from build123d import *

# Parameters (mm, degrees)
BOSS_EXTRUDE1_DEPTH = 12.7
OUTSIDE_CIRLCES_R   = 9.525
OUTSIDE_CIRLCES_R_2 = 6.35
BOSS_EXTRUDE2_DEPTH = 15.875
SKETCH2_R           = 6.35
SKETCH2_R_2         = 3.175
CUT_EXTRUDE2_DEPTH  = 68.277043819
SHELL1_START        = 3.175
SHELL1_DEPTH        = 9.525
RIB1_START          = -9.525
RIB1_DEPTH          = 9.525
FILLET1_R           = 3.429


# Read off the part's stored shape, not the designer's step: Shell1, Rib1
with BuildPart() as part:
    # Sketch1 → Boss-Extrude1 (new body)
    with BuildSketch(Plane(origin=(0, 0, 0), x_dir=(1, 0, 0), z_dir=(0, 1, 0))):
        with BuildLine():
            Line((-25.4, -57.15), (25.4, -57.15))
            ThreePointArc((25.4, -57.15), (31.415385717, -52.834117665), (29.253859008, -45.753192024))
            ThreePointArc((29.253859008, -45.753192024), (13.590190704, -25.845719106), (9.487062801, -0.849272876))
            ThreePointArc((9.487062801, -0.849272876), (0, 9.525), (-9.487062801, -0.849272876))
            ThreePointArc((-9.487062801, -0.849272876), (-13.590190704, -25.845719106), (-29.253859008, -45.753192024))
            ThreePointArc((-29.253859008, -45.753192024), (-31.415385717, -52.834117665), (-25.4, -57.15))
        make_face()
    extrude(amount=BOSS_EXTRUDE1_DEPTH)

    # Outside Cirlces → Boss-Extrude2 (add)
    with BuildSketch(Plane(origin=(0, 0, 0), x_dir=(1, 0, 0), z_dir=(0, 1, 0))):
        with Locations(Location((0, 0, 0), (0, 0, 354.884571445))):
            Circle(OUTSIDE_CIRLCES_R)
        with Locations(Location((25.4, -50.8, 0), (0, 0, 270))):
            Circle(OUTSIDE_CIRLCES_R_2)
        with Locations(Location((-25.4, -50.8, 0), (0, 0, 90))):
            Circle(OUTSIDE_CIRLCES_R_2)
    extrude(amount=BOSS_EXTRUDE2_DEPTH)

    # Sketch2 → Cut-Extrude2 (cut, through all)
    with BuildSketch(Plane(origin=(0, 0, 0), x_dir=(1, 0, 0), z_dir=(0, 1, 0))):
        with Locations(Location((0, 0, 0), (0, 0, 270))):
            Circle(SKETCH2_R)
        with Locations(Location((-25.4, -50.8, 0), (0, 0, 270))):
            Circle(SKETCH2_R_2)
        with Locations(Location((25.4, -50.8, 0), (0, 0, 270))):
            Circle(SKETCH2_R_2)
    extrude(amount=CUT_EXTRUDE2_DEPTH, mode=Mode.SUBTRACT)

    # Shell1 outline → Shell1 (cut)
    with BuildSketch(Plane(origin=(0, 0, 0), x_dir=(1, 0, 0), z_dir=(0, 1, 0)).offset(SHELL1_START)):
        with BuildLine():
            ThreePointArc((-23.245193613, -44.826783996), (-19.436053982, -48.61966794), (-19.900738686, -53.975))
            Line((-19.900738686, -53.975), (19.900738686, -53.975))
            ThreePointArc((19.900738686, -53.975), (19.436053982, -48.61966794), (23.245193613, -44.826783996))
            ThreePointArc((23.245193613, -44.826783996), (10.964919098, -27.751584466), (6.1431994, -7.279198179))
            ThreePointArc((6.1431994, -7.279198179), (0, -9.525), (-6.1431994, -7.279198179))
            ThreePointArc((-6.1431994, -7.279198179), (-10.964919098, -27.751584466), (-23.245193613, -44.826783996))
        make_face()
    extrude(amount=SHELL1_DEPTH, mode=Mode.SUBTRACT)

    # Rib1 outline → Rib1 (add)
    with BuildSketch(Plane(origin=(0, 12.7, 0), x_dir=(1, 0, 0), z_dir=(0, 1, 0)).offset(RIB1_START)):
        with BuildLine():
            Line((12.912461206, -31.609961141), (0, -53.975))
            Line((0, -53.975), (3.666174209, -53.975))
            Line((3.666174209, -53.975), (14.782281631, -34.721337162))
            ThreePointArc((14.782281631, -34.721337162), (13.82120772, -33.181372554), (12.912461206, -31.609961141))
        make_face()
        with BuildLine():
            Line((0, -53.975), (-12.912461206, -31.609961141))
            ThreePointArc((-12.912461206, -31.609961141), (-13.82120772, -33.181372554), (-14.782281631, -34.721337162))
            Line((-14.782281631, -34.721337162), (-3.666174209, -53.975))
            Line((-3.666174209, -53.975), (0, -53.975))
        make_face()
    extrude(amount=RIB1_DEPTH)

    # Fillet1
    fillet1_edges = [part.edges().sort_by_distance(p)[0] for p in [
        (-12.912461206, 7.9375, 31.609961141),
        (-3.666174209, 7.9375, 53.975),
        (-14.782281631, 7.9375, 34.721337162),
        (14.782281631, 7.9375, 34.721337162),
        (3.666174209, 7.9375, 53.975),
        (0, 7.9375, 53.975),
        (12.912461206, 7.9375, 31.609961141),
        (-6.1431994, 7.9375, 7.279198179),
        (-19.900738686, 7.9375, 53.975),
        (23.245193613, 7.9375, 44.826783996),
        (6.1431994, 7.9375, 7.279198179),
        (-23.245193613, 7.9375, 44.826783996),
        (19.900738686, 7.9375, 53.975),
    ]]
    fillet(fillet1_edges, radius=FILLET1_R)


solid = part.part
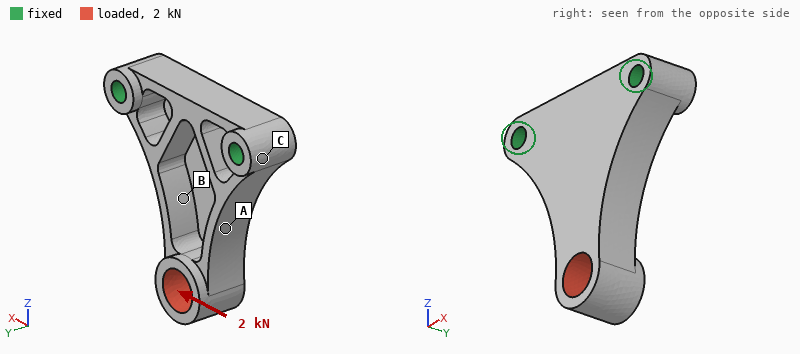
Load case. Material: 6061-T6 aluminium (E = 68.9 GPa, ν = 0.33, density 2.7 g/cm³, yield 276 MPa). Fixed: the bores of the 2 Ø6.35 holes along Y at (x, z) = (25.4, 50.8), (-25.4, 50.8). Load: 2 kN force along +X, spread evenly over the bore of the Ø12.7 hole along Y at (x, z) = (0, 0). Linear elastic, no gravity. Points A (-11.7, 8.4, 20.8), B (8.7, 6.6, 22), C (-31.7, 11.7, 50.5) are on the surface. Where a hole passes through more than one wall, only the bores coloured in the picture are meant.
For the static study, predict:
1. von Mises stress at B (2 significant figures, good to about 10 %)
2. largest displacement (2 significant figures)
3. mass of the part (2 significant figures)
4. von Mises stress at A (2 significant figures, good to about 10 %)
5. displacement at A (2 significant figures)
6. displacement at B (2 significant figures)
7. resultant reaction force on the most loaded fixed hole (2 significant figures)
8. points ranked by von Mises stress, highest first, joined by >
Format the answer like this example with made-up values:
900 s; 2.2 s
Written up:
33 MPa; 0.17 mm; 45 g; 93 MPa; 0.038 mm; 0.030 mm; 2.2 kN; A > B > C
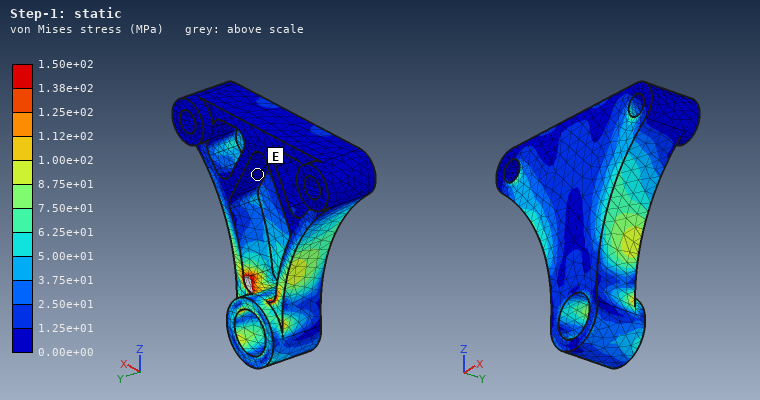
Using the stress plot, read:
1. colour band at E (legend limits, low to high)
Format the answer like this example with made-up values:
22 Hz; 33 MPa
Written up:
0.00e+00 to 1.25e+01 MPa
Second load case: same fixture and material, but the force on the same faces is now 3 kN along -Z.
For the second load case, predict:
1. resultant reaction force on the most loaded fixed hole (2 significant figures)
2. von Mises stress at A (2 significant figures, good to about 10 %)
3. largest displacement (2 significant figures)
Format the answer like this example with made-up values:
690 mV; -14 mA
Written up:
1.7 kN; 65 MPa; 0.15 mm
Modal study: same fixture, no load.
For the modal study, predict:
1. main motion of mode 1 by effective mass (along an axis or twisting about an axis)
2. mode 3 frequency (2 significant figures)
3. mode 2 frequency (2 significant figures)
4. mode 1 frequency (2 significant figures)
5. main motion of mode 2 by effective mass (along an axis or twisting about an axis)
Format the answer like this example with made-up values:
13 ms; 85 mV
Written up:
along Y; 9600 Hz; 6500 Hz; 2800 Hz; along X
